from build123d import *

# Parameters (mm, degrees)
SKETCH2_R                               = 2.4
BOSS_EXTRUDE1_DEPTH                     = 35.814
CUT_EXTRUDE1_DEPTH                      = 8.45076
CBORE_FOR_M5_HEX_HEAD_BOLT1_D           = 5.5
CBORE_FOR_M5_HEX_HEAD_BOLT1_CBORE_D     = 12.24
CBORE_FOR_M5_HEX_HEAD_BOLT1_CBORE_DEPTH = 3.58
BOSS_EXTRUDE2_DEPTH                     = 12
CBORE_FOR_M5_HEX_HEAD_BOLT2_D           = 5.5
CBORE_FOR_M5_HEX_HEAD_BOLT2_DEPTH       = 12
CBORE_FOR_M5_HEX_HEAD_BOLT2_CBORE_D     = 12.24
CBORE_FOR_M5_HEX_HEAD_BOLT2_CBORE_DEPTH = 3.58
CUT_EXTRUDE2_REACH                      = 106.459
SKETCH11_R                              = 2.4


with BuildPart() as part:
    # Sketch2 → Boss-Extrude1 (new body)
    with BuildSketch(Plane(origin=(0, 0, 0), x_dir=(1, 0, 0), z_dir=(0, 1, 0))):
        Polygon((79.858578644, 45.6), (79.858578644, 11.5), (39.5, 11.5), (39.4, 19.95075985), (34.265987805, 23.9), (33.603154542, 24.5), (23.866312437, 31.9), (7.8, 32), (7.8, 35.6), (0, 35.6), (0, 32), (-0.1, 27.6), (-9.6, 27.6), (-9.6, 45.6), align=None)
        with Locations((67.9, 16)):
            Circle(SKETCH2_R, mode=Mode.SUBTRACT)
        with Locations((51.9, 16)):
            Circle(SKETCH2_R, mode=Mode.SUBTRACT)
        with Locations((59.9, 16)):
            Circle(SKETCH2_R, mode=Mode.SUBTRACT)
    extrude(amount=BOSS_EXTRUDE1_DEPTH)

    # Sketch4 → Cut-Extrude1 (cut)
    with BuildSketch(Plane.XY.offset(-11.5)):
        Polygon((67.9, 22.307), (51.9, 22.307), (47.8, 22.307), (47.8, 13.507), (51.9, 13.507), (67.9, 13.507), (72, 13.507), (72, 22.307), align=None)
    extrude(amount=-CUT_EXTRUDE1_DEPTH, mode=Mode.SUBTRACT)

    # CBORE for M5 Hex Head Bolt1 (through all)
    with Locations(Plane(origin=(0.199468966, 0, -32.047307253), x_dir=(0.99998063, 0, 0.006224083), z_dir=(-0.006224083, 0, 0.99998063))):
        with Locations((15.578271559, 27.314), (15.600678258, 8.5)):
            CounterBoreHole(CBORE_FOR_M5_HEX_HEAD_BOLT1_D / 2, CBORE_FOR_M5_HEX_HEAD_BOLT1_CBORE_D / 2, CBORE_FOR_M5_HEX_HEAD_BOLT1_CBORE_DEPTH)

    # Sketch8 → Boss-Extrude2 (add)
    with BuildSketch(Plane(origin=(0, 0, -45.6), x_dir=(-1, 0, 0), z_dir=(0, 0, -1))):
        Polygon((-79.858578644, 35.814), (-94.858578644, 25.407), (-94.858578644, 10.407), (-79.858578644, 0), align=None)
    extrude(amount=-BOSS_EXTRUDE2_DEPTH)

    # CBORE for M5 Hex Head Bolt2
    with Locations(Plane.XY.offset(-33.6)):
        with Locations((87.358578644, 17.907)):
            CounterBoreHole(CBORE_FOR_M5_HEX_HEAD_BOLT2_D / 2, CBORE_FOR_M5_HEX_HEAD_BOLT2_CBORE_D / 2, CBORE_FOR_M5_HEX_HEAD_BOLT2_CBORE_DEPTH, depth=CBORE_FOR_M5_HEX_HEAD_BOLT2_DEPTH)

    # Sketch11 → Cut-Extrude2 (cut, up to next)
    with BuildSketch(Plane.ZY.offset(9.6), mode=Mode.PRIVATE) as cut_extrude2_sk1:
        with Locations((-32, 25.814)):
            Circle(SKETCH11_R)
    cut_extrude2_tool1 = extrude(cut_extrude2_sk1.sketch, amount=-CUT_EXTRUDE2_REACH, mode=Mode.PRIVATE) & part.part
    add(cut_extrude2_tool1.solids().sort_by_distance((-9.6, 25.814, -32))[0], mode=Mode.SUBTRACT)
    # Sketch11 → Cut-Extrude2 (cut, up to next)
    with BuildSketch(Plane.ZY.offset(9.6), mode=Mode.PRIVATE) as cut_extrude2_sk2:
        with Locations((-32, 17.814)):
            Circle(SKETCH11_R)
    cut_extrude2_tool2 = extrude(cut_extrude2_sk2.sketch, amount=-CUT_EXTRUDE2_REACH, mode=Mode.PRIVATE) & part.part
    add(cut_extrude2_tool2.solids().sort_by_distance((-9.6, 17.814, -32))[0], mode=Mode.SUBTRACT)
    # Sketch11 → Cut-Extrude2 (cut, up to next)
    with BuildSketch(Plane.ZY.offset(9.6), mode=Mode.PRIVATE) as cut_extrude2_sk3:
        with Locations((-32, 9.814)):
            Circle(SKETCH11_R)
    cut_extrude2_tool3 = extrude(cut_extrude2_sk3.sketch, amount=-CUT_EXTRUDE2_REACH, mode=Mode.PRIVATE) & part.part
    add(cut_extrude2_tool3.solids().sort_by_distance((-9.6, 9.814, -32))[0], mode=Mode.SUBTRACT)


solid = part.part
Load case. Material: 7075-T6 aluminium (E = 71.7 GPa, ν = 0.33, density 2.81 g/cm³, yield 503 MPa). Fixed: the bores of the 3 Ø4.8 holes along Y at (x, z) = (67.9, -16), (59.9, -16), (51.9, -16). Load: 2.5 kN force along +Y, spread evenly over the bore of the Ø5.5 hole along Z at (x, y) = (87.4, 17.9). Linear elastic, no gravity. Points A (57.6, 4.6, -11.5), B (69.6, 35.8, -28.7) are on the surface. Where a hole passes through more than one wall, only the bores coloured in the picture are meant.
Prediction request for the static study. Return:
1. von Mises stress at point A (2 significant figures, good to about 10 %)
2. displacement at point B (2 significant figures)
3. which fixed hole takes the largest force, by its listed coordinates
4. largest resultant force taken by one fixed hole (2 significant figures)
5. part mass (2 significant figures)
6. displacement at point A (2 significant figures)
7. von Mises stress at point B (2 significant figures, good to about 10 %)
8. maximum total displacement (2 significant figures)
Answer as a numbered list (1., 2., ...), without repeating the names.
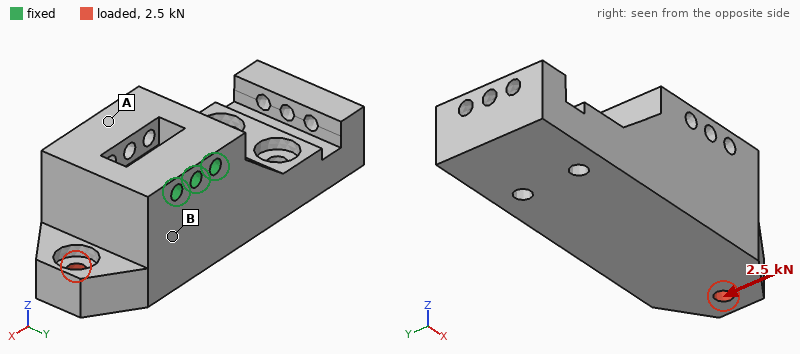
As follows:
1. 7.1 MPa
2. 15 µm
3. (67.9, -16)
4. 3.0 kN
5. 210 g
6. 24 µm
7. 21 MPa
8. 55 µm
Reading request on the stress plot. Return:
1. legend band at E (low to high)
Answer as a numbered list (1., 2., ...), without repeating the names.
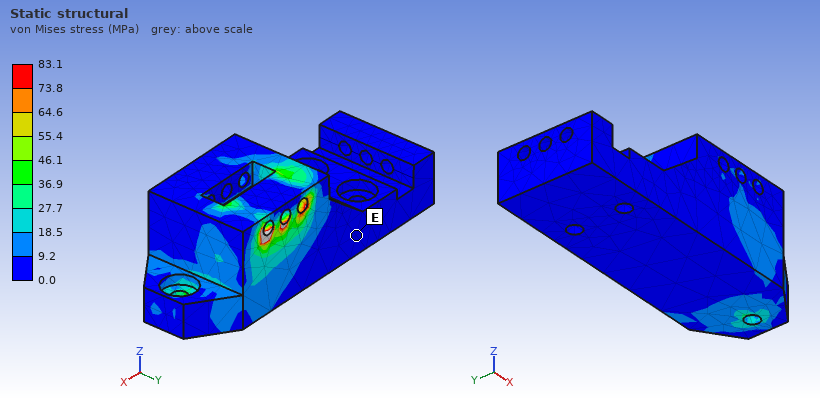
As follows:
1. 0.0 to 9.2 MPa
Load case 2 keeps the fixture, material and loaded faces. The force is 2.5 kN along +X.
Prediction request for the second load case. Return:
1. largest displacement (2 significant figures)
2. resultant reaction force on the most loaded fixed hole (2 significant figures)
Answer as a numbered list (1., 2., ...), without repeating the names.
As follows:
1. 28 µm
2. 3.2 kN
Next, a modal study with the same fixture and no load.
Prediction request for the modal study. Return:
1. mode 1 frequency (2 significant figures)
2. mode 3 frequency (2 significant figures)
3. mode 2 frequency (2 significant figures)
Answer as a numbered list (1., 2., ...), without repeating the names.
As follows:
1. 3000 Hz
2. 4900 Hz
3. 3500 Hz
